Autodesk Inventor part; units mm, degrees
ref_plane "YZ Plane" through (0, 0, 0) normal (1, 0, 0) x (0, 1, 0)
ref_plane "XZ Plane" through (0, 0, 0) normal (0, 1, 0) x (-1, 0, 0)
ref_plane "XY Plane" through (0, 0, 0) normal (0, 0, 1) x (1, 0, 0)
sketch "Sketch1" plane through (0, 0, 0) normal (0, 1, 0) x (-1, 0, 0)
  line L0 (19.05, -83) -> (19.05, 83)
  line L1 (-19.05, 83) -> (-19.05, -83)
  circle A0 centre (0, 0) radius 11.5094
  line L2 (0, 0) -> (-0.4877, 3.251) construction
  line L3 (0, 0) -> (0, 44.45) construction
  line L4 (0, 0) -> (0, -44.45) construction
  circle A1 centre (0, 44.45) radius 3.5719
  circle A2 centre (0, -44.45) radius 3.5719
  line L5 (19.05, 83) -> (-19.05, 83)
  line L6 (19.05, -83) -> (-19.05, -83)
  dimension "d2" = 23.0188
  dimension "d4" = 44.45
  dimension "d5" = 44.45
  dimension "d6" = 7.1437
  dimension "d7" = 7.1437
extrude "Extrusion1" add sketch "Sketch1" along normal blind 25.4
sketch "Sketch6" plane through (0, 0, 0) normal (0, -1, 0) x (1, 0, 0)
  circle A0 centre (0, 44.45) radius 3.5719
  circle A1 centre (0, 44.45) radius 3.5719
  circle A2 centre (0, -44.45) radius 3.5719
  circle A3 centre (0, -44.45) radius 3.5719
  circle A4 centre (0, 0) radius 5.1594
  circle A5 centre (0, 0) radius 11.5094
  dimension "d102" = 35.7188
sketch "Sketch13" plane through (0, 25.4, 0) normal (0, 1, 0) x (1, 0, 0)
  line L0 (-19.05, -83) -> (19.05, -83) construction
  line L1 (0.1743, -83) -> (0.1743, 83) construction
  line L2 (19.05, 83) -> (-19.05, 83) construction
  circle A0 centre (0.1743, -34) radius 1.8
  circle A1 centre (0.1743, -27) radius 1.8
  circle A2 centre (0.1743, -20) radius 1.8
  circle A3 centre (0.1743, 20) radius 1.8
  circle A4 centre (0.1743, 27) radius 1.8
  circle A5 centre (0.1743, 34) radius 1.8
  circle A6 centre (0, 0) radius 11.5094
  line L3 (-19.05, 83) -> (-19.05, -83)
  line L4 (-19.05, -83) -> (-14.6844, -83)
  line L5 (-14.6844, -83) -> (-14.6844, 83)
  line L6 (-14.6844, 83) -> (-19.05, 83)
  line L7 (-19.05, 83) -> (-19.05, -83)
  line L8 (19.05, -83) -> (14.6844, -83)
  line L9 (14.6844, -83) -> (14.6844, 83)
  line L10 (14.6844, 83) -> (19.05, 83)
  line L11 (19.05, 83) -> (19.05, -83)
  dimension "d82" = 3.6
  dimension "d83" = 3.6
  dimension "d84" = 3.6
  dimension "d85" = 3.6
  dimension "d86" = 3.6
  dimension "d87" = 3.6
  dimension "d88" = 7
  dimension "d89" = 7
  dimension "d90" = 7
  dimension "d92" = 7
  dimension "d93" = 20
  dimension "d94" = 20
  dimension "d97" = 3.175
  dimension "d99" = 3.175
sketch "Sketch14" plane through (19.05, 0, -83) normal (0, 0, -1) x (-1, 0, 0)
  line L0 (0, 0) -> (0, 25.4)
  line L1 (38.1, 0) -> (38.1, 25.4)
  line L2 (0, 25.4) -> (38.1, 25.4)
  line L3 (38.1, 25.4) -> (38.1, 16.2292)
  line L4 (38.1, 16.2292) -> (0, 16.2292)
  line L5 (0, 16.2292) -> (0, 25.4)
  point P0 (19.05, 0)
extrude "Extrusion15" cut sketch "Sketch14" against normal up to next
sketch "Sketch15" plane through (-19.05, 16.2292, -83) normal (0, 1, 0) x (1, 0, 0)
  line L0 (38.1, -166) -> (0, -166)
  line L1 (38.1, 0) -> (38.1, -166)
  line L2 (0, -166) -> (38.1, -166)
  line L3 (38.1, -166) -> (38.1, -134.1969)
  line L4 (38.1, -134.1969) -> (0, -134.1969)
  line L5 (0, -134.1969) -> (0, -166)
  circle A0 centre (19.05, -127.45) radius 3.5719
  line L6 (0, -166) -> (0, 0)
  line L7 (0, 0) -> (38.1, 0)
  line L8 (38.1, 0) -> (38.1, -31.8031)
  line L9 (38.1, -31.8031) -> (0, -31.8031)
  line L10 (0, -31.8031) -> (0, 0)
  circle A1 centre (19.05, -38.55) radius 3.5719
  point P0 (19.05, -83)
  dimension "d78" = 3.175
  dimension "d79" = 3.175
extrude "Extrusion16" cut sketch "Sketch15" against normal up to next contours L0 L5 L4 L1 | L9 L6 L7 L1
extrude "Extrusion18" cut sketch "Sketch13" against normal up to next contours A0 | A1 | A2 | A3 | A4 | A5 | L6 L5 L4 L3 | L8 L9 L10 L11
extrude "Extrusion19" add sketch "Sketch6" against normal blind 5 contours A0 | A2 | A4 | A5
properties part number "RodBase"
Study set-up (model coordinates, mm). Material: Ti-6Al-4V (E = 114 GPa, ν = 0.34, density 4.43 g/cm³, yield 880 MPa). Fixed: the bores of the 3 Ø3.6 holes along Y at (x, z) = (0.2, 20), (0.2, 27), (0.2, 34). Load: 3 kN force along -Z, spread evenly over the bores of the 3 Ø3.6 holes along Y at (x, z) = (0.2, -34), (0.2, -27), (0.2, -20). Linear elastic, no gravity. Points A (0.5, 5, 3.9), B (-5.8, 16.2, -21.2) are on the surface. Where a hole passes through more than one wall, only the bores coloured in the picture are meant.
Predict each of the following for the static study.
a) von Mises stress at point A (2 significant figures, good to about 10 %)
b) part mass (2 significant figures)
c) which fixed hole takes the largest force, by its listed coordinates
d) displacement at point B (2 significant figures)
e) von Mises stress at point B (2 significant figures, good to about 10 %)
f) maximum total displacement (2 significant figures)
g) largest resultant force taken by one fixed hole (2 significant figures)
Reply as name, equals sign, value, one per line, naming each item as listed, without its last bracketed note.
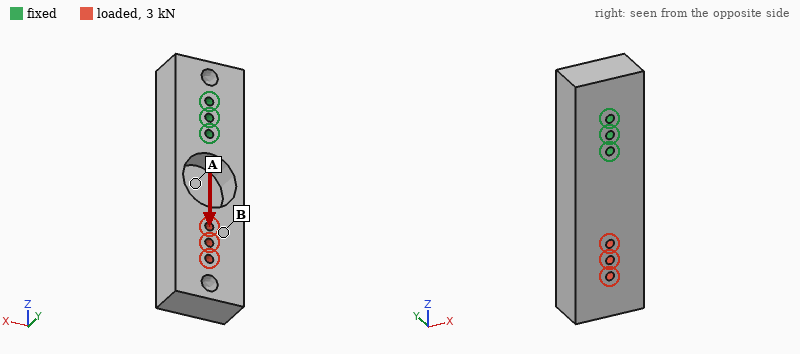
von Mises stress at point A = 17 MPa
part mass = 190 g
which fixed hole takes the largest force, by its listed coordinates = (0.2, 20)
displacement at point B = 14 µm
von Mises stress at point B = 6.8 MPa
maximum total displacement = 26 µm
largest resultant force taken by one fixed hole = 1.5 kN
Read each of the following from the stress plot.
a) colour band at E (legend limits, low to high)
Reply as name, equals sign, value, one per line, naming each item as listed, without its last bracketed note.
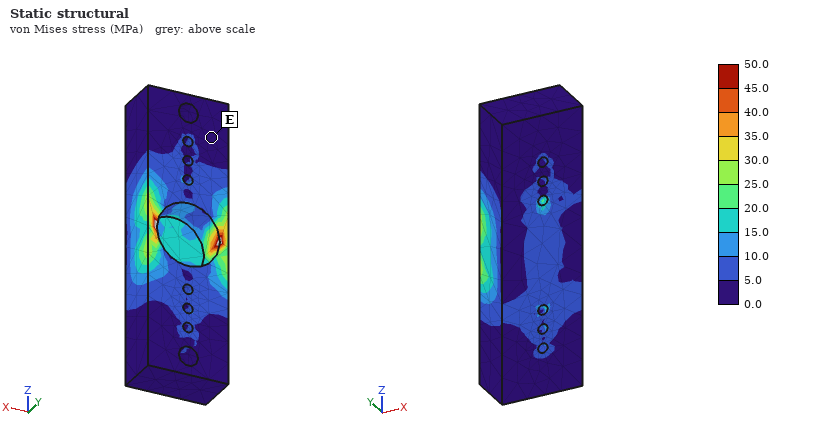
colour band at E = 0.0 to 5.0 MPa
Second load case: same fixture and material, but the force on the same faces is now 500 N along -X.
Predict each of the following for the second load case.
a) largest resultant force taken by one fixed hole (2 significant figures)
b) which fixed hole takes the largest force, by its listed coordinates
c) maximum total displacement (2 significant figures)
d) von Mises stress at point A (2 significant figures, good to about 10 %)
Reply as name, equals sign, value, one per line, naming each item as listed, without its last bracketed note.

largest resultant force taken by one fixed hole = 1.8 kN
which fixed hole takes the largest force, by its listed coordinates = (0.2, 20)
maximum total displacement = 25 µm
von Mises stress at point A = 8.9 MPa
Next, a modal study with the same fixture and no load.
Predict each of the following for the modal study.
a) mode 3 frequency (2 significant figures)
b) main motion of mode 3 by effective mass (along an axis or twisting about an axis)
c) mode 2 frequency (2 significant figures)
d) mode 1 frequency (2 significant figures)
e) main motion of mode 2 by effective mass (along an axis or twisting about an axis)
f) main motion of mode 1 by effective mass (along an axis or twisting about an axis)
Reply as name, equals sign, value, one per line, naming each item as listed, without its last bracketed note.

mode 3 frequency = 6200 Hz
main motion of mode 3 by effective mass = twisting about Z
mode 2 frequency = 2800 Hz
mode 1 frequency = 1800 Hz
main motion of mode 2 by effective mass = along X
main motion of mode 1 by effective mass = along Y
